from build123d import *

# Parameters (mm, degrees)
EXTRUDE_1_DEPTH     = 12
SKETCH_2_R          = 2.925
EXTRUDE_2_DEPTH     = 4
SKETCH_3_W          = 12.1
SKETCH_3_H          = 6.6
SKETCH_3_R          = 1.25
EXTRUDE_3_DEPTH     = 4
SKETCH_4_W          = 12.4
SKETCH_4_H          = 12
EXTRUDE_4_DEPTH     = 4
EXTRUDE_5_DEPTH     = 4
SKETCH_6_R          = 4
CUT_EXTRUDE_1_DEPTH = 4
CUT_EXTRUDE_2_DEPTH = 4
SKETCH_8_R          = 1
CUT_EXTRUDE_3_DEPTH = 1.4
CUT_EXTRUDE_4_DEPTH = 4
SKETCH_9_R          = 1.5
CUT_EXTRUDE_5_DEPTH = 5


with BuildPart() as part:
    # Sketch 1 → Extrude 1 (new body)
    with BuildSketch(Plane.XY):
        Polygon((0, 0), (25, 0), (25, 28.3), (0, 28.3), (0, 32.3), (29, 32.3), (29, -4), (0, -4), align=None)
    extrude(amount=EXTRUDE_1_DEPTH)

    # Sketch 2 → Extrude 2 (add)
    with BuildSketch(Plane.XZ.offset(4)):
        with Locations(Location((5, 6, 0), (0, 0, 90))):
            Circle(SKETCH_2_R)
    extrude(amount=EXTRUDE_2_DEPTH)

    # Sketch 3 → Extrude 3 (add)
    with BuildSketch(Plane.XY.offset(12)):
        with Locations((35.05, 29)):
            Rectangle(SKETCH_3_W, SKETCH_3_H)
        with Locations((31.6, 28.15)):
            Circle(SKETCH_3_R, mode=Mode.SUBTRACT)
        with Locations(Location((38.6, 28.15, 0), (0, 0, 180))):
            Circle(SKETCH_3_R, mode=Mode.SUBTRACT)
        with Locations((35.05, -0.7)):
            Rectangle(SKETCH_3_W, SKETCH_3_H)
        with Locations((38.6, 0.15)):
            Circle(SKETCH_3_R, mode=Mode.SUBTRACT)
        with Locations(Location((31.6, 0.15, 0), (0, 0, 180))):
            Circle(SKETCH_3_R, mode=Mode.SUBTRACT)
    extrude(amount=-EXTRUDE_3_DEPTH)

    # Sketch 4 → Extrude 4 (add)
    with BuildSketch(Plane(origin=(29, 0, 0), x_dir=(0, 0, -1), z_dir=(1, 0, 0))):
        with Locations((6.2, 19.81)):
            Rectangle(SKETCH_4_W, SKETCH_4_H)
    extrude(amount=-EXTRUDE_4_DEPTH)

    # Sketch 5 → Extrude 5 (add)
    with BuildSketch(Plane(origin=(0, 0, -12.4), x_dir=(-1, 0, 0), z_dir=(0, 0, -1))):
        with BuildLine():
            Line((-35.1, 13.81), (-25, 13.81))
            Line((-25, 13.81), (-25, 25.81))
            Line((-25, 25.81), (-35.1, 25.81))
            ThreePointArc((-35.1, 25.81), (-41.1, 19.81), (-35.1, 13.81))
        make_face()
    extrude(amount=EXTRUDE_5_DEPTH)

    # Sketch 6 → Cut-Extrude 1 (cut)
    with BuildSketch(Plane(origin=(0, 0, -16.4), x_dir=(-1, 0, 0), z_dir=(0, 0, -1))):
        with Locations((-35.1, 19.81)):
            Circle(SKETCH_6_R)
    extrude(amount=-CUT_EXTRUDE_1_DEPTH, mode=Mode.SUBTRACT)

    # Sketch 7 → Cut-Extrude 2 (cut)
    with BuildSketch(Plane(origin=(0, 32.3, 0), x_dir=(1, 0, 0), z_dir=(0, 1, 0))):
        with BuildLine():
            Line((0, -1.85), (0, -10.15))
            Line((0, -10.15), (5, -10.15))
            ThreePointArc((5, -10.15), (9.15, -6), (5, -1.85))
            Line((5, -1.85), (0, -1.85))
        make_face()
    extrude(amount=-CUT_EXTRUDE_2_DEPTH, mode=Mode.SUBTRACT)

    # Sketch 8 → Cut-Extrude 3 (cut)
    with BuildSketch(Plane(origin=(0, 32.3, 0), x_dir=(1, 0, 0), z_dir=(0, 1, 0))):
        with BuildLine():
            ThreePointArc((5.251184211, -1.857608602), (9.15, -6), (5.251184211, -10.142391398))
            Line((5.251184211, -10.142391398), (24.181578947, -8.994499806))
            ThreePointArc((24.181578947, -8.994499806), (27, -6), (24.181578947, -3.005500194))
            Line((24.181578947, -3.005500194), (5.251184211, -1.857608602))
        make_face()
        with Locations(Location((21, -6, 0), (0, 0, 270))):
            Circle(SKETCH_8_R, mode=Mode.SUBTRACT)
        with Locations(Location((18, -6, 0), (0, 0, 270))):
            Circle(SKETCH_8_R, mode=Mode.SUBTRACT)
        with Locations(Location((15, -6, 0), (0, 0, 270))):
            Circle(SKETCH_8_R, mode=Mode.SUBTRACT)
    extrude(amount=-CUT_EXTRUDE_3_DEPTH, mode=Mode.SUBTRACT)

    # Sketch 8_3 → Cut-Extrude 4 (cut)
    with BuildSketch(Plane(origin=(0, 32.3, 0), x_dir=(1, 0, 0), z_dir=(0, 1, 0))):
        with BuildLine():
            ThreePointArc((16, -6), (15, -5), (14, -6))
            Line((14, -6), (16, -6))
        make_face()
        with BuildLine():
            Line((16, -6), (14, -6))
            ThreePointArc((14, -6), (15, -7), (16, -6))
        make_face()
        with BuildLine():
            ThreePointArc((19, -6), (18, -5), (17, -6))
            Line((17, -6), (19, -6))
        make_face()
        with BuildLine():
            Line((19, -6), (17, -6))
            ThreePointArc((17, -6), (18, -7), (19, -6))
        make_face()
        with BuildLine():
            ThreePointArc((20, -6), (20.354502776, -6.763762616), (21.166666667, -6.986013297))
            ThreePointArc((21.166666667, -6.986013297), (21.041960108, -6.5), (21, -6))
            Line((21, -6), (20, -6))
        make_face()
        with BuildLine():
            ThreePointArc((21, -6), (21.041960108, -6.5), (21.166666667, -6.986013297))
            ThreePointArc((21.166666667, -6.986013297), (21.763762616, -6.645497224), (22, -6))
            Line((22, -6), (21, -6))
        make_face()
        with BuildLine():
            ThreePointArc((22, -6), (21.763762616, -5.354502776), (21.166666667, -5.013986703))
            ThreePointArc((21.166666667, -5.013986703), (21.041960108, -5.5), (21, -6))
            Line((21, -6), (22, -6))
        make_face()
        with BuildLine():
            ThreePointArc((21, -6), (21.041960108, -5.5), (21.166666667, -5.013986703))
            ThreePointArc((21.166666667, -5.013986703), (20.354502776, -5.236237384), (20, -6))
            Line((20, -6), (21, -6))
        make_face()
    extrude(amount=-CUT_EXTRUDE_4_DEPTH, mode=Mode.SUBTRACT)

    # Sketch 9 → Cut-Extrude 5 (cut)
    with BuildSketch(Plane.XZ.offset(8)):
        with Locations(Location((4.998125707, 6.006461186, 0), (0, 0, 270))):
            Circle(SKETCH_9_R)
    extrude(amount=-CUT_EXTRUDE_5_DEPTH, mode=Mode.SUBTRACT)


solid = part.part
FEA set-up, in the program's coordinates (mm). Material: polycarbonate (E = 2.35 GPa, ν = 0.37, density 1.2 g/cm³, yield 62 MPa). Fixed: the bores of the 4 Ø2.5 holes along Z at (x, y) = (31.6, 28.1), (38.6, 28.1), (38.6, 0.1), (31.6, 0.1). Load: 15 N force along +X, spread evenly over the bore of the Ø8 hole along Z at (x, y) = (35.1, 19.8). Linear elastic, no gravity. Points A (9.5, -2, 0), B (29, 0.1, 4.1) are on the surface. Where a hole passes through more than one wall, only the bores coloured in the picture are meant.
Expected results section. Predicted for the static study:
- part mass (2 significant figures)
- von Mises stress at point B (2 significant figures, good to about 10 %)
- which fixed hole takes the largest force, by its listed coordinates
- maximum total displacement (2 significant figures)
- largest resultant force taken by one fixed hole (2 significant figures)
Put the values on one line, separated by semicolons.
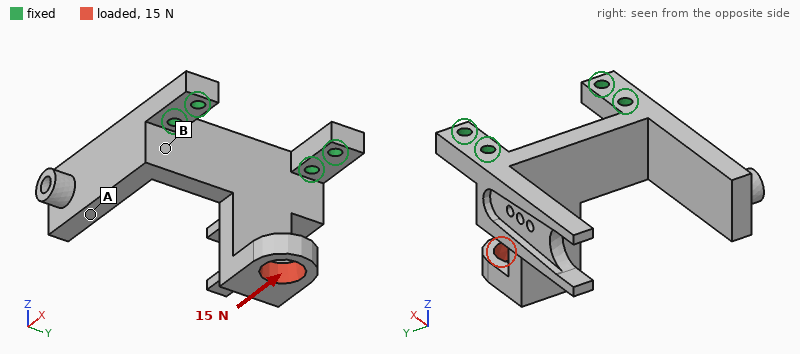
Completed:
6.5 g; 2.3 MPa; (31.6, 28.1); 0.76 mm; 13 N
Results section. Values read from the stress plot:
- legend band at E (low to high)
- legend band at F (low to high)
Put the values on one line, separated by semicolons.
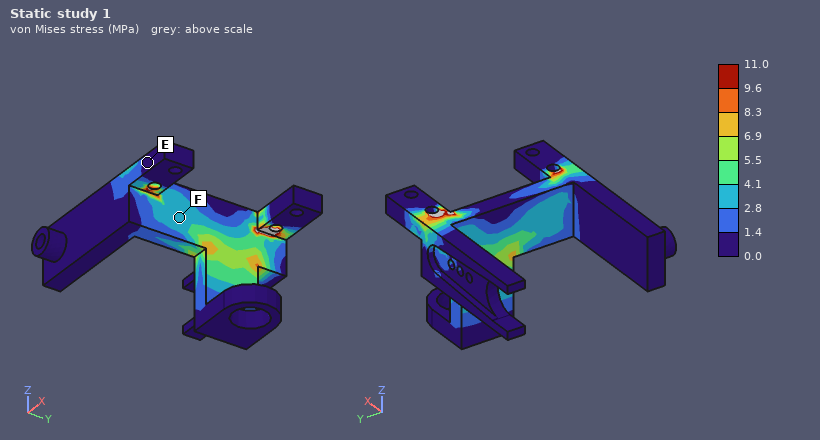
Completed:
0.0 to 1.4 MPa; 2.8 to 4.1 MPa
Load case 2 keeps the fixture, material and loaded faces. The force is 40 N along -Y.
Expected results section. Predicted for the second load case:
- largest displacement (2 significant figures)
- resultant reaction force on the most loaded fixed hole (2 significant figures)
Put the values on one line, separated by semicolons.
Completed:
0.65 mm; 46 N
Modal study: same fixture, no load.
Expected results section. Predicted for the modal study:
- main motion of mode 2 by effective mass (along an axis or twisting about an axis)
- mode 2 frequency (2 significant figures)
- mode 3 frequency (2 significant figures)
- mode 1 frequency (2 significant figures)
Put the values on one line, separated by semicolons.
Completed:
along Y; 960 Hz; 1100 Hz; 730 Hz
